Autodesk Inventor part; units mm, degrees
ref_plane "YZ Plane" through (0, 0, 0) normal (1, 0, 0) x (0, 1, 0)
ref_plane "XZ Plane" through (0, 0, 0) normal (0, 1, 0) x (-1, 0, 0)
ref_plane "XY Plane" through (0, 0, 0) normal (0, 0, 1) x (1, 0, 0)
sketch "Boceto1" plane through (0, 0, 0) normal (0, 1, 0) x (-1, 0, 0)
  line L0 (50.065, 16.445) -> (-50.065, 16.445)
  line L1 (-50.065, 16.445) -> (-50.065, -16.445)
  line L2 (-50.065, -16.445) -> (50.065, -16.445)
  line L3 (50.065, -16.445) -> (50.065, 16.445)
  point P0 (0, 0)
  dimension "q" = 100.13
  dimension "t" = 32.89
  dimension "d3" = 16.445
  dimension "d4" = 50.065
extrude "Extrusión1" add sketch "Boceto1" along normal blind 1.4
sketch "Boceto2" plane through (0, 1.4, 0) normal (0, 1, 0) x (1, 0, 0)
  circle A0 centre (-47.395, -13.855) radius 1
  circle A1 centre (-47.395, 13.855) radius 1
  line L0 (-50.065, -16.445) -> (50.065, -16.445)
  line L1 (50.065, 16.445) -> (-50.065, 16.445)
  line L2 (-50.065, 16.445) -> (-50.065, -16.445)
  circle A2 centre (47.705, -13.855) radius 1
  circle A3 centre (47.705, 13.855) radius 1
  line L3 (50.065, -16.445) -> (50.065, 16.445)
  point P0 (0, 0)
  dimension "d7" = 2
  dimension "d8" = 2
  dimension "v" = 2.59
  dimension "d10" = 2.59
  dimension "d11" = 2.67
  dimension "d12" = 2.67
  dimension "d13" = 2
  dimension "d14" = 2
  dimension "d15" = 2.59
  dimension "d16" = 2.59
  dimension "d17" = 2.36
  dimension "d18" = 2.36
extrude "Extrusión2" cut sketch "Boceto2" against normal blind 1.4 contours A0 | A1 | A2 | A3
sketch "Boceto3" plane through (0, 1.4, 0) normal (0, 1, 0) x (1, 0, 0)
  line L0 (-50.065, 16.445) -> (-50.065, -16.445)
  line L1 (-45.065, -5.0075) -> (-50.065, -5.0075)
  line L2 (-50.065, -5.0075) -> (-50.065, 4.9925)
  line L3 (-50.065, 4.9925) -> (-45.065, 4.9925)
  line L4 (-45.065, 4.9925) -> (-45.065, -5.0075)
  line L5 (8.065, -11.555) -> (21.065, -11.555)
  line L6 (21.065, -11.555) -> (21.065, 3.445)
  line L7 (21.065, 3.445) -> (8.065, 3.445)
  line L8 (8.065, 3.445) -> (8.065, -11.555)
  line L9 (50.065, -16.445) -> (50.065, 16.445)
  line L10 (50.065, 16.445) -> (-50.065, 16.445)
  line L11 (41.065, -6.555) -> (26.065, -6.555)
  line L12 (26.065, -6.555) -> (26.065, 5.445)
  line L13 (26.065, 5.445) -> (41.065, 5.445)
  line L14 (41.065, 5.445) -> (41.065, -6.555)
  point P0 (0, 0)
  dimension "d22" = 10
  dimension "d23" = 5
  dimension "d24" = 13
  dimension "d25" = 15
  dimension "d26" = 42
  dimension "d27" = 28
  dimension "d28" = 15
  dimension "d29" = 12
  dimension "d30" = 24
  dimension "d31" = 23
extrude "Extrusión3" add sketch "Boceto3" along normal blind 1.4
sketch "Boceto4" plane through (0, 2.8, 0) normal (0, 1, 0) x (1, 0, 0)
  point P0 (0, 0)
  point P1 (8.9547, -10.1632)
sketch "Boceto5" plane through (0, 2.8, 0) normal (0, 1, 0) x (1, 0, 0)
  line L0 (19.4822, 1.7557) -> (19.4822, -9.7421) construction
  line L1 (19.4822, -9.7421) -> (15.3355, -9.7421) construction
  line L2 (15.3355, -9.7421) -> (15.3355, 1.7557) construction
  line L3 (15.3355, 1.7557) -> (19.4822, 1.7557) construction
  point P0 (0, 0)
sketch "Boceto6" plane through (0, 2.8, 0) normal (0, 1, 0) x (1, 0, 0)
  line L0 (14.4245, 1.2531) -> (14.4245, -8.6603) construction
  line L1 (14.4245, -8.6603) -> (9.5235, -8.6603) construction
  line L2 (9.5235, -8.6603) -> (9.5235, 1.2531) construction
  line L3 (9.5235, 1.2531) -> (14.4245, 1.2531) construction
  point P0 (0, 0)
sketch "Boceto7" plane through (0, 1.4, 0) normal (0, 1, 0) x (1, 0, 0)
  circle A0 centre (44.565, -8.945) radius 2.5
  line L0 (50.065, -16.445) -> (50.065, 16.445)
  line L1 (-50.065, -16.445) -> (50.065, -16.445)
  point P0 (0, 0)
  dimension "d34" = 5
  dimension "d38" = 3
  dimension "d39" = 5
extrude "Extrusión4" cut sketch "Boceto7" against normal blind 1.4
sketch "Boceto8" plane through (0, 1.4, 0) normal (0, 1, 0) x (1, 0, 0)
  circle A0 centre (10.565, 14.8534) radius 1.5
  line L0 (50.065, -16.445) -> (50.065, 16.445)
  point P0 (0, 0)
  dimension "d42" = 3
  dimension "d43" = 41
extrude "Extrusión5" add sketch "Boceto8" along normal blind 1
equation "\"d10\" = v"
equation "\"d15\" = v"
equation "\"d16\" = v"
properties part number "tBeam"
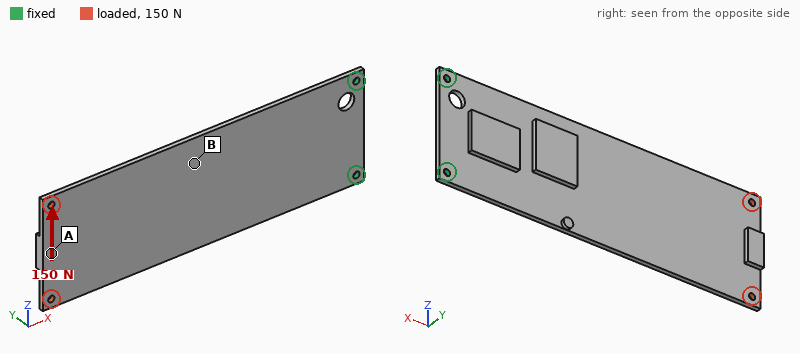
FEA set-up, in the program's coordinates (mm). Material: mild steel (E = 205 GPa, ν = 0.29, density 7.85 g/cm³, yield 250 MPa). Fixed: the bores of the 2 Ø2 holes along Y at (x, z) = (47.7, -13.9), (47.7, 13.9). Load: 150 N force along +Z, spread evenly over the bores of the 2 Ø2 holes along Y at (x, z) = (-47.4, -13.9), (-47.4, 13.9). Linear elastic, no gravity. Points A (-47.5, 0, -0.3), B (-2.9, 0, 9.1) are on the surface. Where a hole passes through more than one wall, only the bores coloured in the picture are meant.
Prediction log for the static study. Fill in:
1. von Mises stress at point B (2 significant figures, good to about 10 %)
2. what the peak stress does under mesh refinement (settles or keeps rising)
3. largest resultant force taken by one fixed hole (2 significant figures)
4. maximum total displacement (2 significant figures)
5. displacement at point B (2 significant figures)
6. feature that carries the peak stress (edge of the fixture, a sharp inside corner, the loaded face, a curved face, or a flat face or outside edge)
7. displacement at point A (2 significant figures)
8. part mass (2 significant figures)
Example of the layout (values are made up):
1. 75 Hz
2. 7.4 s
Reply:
1. 16 MPa
2. keeps rising
3. 520 N
4. 66 µm
5. 23 µm
6. edge of the fixture
7. 60 µm
8. 41 g
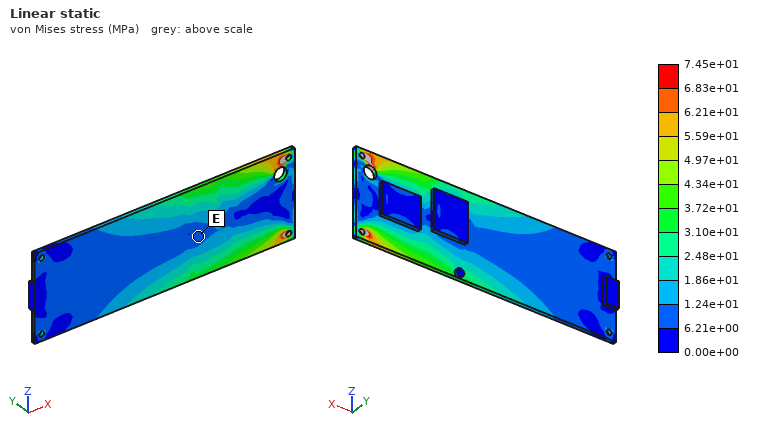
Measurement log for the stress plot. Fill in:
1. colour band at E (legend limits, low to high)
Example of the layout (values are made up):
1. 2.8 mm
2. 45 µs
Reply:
1. 6.21e+00 to 1.24e+01 MPa
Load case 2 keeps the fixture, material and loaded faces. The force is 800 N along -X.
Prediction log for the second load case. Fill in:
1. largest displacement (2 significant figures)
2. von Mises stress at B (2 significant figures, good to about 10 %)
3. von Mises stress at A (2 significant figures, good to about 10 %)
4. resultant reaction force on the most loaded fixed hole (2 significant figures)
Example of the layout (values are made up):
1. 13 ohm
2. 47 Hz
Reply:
1. 57 µm
2. 18 MPa
3. 18 MPa
4. 420 N
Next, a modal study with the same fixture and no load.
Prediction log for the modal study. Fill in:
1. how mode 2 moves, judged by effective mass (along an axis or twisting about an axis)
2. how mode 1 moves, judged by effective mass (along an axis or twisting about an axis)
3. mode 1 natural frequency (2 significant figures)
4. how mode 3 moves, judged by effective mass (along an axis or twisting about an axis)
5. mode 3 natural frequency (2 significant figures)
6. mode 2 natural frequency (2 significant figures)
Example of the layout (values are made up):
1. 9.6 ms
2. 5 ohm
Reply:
1. along Y
2. along Y
3. 130 Hz
4. twisting about X
5. 940 Hz
6. 710 Hz
